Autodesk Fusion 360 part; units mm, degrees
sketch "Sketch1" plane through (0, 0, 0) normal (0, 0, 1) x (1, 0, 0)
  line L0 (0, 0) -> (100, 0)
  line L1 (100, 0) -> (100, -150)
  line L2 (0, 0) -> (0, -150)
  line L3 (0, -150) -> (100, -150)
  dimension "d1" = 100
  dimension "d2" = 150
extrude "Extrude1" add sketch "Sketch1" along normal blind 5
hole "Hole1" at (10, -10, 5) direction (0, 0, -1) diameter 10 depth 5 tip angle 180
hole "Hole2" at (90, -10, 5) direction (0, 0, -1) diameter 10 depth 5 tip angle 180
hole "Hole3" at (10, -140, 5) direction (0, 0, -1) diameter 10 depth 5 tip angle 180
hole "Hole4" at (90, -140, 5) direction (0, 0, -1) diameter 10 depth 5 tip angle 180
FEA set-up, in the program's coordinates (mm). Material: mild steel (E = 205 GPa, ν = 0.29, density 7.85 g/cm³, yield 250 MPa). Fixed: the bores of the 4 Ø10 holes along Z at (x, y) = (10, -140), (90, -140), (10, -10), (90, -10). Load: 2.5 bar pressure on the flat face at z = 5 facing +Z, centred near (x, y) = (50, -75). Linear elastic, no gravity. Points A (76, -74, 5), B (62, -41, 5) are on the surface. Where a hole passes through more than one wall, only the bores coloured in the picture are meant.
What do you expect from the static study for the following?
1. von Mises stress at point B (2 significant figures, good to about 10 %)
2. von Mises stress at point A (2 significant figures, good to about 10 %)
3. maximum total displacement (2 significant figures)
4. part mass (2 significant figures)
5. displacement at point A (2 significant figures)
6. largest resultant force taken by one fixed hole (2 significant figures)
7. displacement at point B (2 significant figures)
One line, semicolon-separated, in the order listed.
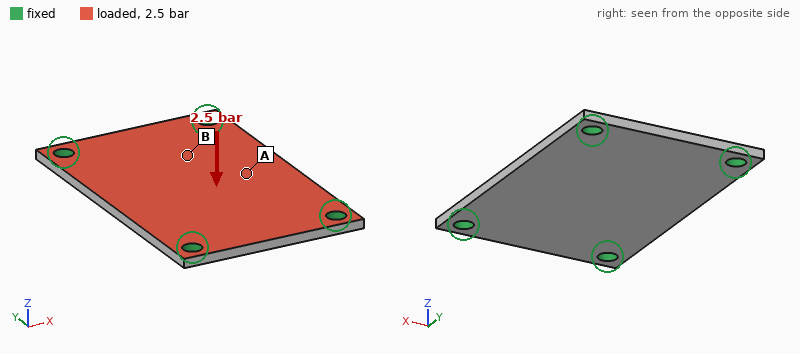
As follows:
18 MPa; 40 MPa; 0.10 mm; 580 g; 0.098 mm; 920 N; 0.065 mm
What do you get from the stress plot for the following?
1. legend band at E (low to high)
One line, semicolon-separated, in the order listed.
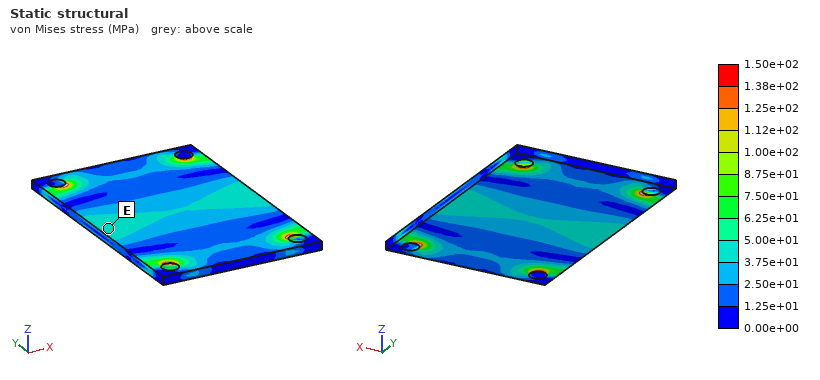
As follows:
3.75e+01 to 5.00e+01 MPa
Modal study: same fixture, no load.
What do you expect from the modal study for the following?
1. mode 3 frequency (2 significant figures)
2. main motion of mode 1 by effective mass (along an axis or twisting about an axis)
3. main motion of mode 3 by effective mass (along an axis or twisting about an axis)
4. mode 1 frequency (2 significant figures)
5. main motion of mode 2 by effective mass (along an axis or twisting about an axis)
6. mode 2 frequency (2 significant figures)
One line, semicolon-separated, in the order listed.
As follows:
3700 Hz; along Z; twisting about X; 1500 Hz; twisting about Y; 2200 Hz
